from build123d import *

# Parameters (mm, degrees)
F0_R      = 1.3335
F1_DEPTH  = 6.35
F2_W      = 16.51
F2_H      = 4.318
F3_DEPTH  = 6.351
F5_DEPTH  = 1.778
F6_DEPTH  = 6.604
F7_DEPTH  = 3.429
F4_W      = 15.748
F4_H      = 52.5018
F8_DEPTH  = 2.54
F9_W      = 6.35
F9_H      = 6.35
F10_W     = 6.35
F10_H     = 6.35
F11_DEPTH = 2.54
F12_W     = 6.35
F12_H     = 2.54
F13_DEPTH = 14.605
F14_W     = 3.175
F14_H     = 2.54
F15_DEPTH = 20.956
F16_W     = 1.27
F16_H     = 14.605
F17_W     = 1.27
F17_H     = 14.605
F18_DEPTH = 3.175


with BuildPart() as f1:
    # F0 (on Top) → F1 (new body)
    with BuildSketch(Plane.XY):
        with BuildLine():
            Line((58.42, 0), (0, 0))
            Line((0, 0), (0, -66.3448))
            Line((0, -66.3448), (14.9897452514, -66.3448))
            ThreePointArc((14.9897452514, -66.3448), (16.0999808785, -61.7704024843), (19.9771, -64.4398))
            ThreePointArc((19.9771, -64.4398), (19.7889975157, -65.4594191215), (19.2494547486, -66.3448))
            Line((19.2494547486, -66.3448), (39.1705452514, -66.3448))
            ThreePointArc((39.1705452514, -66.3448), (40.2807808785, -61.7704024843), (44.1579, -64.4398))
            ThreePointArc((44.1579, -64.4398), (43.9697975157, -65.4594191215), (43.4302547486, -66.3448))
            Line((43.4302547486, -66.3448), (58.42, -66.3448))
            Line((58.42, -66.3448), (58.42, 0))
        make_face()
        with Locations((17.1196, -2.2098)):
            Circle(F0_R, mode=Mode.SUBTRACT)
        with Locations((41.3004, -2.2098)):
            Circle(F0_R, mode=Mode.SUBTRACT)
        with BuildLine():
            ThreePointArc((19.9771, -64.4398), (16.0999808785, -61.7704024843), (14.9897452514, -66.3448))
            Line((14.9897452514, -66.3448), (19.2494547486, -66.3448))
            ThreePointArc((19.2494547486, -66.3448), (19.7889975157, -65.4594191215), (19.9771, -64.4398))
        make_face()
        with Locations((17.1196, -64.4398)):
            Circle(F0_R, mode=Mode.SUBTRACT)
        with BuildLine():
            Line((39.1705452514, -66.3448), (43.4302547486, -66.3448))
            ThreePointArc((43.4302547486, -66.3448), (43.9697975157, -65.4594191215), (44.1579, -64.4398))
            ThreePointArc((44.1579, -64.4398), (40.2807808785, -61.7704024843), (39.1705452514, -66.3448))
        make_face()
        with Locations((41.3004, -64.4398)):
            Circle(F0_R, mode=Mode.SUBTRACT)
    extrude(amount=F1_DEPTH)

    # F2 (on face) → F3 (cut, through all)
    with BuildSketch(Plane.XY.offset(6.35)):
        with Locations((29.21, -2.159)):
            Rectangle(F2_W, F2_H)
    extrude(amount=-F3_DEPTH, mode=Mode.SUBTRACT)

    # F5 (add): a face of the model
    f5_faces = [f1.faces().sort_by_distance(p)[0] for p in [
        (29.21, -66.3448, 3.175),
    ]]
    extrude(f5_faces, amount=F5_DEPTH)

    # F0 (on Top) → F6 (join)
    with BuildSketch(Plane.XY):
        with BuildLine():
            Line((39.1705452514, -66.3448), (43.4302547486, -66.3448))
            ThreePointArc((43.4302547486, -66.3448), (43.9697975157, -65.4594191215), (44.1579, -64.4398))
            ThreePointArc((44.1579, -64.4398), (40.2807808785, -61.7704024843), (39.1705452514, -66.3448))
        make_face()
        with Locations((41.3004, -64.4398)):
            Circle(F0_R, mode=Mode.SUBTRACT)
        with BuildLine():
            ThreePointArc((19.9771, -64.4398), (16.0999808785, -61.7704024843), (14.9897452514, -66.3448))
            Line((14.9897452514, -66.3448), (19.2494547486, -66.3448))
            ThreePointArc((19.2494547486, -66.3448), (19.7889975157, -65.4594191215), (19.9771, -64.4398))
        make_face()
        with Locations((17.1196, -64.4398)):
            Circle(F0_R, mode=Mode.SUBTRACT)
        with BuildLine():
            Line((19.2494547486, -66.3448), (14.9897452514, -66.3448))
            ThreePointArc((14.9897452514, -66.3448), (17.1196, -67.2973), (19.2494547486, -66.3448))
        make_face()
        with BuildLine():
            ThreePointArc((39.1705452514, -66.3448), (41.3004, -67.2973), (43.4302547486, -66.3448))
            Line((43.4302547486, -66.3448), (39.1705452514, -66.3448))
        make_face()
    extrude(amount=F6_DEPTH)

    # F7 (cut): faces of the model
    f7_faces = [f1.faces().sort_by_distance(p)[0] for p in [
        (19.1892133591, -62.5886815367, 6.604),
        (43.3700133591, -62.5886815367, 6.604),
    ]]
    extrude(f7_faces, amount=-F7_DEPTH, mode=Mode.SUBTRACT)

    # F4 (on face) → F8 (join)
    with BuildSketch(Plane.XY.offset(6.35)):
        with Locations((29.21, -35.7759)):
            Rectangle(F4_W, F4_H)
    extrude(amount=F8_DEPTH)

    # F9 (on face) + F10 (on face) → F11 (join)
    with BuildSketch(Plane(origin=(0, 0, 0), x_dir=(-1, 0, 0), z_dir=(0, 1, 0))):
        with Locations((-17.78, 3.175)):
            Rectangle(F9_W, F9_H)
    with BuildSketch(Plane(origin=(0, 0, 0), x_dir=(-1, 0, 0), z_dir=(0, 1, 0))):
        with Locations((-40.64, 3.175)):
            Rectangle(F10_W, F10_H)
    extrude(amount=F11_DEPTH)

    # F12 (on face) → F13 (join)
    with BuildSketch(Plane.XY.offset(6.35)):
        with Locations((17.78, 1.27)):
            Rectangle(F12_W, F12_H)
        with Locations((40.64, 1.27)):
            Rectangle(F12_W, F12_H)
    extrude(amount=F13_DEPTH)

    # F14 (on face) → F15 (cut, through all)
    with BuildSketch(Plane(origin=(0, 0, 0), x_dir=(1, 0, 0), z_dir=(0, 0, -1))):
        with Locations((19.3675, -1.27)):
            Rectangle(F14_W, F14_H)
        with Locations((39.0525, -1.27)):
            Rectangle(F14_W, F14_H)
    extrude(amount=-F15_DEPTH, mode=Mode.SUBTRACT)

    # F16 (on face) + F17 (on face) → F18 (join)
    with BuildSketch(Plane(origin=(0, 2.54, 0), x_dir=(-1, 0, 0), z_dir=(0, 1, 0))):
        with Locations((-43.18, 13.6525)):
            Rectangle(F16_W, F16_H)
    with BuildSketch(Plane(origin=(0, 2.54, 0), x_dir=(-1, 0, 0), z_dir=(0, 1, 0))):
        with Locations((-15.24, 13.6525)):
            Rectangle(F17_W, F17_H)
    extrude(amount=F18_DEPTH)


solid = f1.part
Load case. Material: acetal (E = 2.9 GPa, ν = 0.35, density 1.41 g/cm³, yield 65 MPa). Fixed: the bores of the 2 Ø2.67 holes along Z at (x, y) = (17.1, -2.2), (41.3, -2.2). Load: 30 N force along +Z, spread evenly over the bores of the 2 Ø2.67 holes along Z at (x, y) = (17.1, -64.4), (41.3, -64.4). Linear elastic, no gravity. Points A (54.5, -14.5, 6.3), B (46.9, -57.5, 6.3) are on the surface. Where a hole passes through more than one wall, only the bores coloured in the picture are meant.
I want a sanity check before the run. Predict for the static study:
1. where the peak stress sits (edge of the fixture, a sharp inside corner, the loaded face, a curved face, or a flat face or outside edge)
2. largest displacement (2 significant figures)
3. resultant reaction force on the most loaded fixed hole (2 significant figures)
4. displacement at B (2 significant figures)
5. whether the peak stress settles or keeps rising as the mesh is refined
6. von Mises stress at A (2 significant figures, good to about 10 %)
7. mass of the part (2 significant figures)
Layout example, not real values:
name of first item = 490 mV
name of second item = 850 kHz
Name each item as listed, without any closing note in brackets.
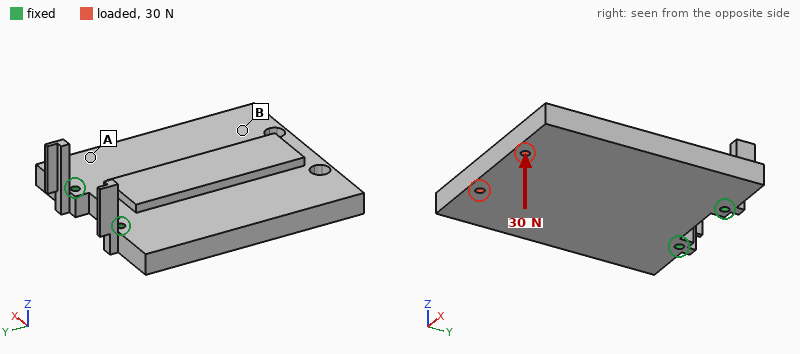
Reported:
where the peak stress sits = edge of the fixture
largest displacement = 0.96 mm
resultant reaction force on the most loaded fixed hole = 18 N
displacement at B = 0.76 mm
whether the peak stress settles or keeps rising as the mesh is refined = keeps rising
von Mises stress at A = 2.9 MPa
mass of the part = 38 g
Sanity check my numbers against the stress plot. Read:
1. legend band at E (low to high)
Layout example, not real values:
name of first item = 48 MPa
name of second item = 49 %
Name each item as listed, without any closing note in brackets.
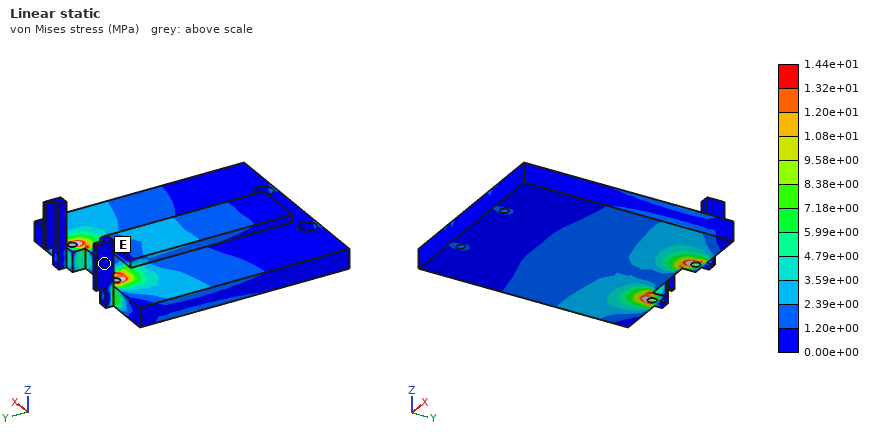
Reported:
legend band at E = 0.00e+00 to 1.20e+00 MPa
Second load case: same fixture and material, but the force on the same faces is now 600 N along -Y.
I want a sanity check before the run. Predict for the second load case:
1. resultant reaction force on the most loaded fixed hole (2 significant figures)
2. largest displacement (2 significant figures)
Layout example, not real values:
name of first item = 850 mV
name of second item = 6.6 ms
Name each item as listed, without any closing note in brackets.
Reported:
resultant reaction force on the most loaded fixed hole = 300 N
largest displacement = 0.73 mm
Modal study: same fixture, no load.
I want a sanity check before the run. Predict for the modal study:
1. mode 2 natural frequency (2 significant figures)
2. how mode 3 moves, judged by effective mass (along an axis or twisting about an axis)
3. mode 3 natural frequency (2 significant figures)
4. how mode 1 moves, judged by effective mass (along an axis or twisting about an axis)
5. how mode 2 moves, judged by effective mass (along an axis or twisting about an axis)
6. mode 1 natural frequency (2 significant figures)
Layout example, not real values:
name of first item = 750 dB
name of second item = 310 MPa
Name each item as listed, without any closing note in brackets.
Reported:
mode 2 natural frequency = 830 Hz
how mode 3 moves, judged by effective mass = along X
mode 3 natural frequency = 1200 Hz
how mode 1 moves, judged by effective mass = along Z
how mode 2 moves, judged by effective mass = twisting about Y
mode 1 natural frequency = 270 Hz
